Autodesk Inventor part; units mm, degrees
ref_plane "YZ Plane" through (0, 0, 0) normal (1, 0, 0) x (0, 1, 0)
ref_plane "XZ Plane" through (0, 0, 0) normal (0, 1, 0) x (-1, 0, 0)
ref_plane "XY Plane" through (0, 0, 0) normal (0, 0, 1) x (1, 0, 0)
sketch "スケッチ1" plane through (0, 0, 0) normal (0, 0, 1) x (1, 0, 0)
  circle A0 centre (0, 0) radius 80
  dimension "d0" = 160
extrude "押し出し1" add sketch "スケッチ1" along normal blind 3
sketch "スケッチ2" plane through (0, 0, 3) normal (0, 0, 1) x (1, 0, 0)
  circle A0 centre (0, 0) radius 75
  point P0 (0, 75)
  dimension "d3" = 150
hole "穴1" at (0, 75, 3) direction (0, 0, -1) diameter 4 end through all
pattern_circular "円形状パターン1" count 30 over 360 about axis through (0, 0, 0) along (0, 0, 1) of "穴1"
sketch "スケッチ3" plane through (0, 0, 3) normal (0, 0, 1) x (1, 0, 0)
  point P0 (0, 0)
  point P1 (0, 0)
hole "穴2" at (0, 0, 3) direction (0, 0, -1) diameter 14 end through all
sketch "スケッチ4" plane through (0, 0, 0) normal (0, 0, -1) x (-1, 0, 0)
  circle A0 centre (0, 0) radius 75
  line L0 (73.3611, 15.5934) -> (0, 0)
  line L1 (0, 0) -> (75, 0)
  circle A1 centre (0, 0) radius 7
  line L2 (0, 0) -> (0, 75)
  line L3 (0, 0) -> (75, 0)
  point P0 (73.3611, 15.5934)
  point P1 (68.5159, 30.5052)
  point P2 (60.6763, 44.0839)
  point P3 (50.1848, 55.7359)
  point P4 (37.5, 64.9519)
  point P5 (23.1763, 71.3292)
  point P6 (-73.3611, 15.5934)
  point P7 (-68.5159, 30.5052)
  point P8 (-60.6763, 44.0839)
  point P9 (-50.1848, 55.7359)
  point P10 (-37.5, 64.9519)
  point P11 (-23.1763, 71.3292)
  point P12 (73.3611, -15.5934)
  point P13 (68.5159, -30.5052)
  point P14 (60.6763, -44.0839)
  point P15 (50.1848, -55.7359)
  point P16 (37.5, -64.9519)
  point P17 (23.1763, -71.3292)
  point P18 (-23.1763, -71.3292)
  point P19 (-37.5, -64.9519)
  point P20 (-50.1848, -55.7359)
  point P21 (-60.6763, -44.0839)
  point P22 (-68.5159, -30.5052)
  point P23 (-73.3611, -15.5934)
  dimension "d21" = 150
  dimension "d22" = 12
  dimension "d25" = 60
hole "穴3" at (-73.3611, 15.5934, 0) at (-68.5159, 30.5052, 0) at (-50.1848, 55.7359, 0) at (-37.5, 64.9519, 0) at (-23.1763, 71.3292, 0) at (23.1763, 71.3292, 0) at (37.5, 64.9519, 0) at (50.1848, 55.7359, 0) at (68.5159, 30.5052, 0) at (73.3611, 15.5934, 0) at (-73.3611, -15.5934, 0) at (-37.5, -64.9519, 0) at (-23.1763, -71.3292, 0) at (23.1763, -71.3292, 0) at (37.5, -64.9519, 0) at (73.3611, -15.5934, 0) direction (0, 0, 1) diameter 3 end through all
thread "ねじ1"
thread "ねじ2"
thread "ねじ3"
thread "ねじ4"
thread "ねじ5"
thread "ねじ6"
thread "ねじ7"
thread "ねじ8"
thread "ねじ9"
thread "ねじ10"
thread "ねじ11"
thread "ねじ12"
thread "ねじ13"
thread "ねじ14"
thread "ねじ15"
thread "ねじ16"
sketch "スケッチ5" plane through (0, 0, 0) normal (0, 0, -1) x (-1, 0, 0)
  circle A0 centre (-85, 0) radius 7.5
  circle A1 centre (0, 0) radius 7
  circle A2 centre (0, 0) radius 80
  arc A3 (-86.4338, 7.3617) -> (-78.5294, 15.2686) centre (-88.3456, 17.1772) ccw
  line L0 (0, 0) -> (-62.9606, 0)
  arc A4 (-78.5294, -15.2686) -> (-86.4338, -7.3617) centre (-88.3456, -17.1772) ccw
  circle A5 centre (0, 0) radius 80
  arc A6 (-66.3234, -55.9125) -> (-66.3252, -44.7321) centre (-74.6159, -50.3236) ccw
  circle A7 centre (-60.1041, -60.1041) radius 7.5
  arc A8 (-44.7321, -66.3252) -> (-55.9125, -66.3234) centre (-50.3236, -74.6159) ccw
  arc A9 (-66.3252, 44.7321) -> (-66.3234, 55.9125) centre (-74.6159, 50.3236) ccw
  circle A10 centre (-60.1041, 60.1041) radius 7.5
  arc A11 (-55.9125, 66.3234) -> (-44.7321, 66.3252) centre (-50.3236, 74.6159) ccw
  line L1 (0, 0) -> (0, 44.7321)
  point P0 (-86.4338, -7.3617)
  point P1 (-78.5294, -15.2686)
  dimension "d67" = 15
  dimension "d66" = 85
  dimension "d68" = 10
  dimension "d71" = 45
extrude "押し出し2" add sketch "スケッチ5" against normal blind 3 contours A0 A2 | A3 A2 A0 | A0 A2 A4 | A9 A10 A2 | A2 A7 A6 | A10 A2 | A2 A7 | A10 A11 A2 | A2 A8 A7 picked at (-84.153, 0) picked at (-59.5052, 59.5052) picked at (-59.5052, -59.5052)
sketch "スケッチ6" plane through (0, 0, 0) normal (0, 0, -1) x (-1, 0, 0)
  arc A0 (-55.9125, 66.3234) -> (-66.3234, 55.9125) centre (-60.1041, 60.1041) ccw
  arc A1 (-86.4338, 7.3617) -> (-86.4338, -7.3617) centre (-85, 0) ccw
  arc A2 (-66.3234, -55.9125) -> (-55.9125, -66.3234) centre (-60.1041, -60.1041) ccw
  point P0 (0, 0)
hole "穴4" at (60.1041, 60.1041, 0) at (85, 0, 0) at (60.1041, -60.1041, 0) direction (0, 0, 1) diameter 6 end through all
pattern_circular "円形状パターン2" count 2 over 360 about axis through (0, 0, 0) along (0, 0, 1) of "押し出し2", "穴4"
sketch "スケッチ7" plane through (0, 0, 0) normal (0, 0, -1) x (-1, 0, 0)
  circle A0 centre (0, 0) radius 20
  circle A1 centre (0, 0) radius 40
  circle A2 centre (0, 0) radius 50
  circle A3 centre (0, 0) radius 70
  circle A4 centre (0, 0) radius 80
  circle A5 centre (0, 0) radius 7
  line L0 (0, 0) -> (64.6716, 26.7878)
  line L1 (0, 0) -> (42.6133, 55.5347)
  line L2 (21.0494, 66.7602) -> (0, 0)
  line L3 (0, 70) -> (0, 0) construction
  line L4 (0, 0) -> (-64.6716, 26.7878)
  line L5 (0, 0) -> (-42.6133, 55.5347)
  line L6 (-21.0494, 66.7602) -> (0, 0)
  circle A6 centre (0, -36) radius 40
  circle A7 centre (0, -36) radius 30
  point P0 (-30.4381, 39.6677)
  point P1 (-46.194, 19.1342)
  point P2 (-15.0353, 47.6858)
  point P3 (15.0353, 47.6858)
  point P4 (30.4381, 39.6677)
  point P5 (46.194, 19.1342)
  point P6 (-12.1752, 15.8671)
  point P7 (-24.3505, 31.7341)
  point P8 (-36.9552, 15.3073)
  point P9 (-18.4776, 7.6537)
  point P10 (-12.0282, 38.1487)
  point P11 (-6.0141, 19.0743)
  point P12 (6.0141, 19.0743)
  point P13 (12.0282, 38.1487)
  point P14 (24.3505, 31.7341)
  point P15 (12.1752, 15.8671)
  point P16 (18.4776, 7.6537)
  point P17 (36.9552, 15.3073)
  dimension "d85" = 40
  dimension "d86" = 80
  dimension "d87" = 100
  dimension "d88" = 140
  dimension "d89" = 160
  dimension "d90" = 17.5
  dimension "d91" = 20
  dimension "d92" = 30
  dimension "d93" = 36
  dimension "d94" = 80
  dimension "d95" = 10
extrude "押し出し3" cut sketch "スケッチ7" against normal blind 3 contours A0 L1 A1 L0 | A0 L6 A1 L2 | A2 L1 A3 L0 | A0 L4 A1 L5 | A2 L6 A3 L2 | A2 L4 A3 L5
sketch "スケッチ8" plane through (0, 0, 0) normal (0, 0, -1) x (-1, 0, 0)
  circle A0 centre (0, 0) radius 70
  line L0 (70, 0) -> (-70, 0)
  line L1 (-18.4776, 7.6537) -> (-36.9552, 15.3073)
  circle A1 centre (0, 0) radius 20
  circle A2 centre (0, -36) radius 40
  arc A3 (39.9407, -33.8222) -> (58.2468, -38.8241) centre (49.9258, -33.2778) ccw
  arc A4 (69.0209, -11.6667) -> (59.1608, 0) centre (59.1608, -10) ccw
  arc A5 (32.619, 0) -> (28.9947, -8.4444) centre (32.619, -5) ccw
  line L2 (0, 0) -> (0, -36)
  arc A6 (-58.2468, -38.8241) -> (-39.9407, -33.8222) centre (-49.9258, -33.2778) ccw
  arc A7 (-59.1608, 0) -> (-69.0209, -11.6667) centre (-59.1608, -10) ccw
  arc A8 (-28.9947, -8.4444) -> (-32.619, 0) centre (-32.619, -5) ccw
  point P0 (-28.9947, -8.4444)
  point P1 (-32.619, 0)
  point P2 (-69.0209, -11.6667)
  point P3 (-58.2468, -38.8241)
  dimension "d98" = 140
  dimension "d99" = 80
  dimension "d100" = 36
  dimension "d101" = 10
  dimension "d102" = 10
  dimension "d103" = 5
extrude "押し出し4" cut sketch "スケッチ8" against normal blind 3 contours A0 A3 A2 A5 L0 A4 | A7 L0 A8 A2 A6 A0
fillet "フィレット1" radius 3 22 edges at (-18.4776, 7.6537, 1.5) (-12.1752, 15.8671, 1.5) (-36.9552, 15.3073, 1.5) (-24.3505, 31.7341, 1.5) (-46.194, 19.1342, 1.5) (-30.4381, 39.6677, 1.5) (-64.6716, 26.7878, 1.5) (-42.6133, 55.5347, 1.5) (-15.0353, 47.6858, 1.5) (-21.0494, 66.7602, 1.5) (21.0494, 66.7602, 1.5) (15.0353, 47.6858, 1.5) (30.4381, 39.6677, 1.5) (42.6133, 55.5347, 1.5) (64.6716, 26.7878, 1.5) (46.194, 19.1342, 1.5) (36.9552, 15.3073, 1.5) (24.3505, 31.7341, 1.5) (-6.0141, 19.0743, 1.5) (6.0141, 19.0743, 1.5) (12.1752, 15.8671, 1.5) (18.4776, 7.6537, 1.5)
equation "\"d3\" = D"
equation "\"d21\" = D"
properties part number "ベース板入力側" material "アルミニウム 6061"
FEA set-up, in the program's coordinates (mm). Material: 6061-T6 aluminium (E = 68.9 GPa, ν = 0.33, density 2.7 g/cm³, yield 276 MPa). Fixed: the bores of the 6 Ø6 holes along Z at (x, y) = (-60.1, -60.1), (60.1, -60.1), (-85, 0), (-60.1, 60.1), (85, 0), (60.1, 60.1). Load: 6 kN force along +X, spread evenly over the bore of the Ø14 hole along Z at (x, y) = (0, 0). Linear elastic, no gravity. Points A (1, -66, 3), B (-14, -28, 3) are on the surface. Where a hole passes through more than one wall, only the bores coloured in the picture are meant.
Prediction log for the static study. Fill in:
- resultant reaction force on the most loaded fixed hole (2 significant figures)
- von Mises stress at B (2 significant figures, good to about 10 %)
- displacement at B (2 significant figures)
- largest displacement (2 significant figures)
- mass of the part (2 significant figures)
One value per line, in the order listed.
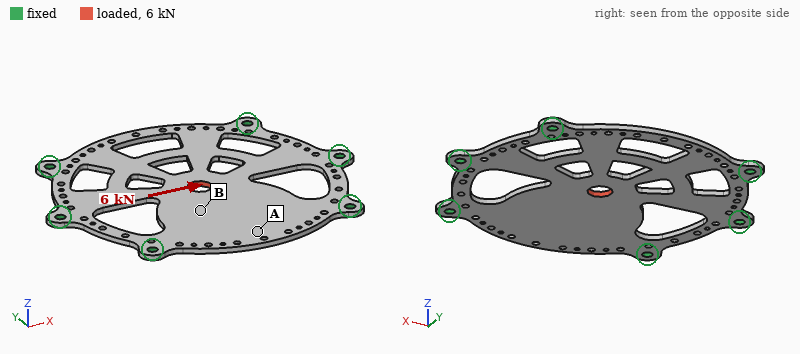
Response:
1.4 kN
20 MPa
23 µm
48 µm
120 g
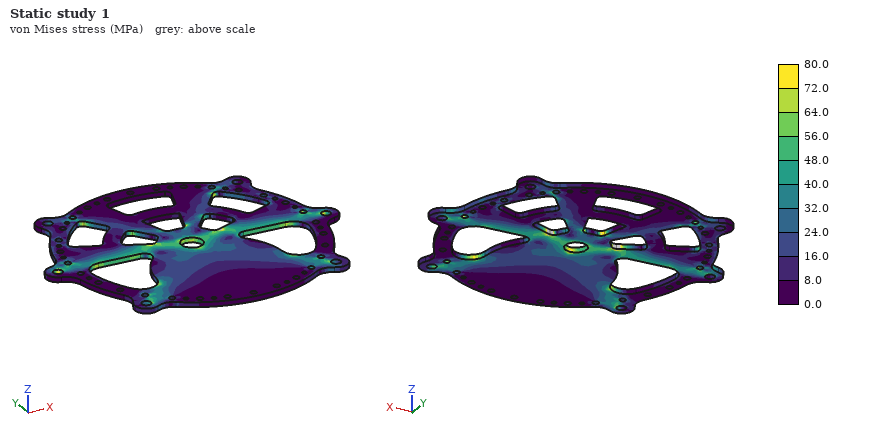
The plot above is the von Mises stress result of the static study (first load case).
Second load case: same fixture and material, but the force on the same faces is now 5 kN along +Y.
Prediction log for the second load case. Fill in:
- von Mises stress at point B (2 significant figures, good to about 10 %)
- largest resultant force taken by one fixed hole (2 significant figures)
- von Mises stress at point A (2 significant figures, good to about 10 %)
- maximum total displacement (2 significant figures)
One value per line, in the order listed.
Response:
19 MPa
1.7 kN
8.8 MPa
56 µm
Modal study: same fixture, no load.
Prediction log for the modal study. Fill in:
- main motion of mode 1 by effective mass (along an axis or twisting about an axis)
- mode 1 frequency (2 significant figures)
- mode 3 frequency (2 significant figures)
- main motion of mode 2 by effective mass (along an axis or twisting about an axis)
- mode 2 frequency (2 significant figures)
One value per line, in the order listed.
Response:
along Z
680 Hz
1200 Hz
twisting about X
1000 Hz
